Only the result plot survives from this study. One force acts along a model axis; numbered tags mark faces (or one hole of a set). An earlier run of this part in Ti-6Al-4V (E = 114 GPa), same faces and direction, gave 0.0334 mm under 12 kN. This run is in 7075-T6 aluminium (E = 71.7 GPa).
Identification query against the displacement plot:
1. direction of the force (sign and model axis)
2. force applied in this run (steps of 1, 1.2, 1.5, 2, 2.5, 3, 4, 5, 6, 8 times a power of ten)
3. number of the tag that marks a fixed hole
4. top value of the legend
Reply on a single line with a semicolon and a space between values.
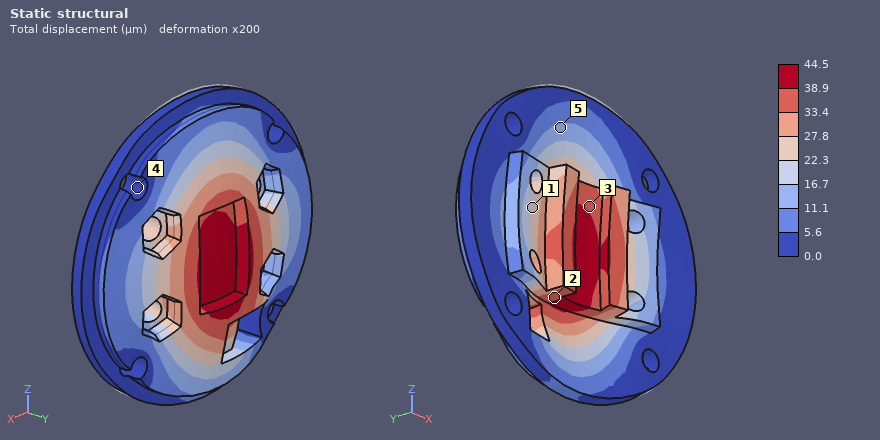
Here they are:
+Y; 10 kN; 4; 44.5 µm
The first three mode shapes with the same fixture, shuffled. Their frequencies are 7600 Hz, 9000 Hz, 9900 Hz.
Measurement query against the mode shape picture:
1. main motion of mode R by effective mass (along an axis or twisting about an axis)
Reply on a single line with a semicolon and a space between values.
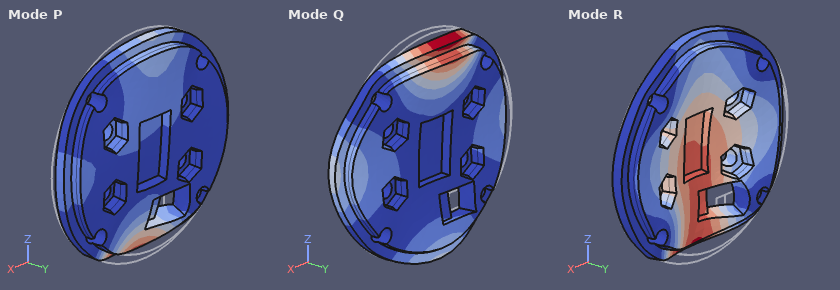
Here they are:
along Y
